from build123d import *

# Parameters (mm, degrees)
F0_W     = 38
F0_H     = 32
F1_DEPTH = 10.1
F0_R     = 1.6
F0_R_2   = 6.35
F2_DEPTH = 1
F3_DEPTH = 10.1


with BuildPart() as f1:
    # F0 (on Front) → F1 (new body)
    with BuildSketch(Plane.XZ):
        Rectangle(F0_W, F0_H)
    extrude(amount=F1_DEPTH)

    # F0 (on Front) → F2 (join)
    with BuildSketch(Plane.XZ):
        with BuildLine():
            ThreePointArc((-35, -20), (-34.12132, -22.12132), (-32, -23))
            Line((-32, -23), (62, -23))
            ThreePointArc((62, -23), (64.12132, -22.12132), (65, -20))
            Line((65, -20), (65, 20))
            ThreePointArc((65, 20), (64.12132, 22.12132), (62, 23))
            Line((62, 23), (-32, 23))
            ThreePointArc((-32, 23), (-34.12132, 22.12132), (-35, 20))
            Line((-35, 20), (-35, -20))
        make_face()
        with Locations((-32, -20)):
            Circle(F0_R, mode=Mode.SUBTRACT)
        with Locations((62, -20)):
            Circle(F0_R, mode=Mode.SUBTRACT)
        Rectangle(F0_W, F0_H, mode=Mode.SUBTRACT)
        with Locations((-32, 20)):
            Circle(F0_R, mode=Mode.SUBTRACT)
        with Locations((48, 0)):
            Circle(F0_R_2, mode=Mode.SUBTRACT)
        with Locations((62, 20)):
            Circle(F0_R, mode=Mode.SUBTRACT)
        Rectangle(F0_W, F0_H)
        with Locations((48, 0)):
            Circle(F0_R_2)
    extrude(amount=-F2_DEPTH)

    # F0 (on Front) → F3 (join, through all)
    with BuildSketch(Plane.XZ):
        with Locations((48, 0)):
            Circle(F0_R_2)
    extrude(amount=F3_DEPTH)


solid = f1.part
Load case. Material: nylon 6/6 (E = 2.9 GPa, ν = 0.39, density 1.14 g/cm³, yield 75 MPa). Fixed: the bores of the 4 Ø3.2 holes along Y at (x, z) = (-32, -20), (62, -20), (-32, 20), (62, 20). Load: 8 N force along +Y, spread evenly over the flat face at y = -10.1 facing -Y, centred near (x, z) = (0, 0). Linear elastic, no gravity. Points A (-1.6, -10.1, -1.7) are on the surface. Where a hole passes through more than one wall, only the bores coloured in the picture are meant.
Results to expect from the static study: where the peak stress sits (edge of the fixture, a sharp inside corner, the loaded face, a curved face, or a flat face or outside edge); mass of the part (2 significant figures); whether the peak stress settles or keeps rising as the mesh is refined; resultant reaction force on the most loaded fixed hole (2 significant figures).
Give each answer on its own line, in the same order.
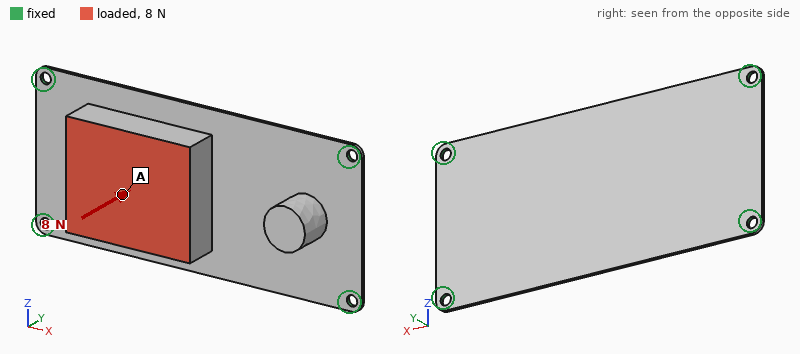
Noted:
edge of the fixture
21 g
keeps rising
3.0 N
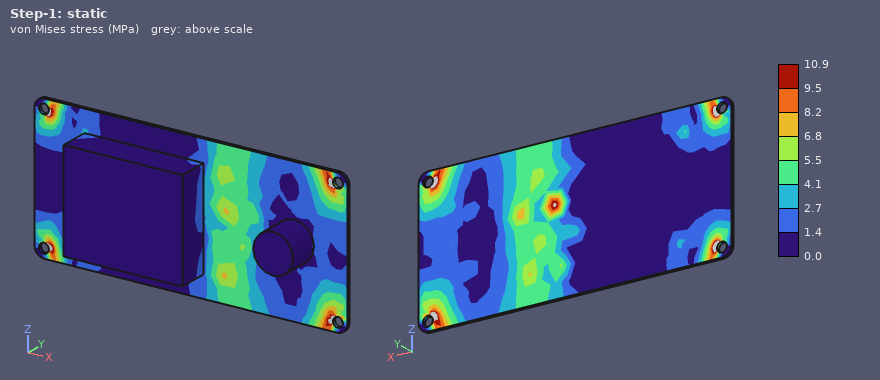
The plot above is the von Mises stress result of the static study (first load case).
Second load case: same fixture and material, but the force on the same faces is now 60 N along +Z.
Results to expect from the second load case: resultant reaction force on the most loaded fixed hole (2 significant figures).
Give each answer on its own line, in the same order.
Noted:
36 N
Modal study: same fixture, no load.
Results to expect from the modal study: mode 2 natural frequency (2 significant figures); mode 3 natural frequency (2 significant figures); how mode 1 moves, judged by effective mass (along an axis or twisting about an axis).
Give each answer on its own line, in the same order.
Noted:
370 Hz
500 Hz
along Y
